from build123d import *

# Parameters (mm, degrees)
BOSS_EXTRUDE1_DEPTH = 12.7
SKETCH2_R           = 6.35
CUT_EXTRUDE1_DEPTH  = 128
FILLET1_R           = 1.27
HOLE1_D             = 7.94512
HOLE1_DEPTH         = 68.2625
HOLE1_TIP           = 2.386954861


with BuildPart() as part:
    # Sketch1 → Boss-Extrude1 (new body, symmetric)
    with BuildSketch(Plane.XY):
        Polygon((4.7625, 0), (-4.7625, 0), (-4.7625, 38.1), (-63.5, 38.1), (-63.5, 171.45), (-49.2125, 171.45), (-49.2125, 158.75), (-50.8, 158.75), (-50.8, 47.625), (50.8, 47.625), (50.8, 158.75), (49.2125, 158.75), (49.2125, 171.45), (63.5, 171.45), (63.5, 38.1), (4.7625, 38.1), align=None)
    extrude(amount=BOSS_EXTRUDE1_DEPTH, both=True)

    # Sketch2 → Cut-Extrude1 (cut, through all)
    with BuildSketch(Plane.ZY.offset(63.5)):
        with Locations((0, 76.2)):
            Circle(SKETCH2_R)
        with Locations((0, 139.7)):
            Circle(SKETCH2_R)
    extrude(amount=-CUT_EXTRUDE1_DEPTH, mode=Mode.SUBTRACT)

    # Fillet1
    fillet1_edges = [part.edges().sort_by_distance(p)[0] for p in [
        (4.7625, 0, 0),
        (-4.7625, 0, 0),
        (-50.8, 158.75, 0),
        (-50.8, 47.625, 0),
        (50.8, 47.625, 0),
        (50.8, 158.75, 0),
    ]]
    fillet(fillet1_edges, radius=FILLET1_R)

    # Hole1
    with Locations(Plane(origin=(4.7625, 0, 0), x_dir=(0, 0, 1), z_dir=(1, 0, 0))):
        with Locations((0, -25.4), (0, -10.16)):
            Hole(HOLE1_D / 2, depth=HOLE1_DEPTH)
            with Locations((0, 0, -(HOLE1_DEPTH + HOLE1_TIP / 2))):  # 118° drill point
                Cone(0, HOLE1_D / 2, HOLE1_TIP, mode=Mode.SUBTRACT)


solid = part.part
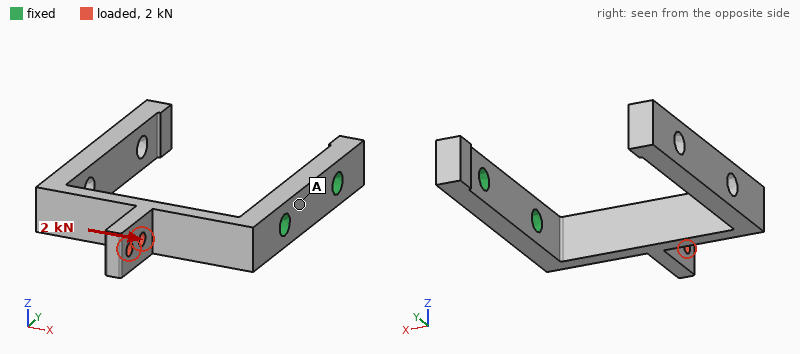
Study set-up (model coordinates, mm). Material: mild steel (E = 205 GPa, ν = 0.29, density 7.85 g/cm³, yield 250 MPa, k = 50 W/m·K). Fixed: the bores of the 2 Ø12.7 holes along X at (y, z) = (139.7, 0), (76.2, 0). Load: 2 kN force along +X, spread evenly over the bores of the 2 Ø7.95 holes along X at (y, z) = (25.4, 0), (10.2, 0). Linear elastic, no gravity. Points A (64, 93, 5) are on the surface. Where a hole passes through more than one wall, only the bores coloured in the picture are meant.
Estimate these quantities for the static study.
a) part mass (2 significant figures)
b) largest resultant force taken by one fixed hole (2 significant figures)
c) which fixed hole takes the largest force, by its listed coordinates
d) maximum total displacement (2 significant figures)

890 g
2.0 kN
(76.2, 0)
1.5 mm
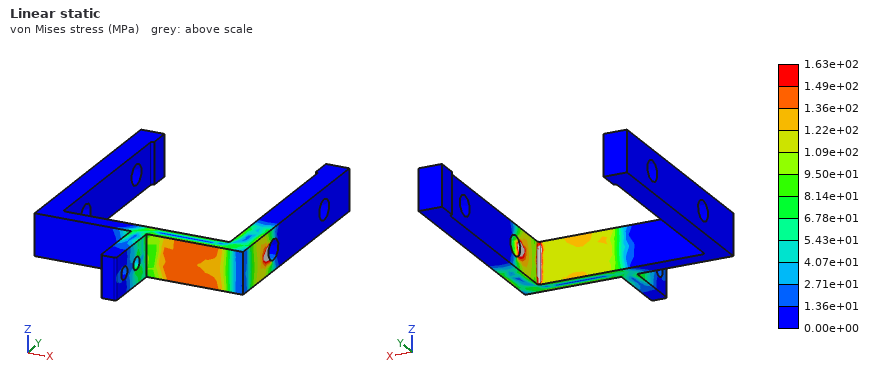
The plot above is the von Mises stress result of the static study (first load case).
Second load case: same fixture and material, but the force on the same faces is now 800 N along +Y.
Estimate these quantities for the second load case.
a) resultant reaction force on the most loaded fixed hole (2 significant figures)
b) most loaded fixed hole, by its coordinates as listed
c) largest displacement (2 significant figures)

790 N
(76.2, 0)
0.74 mm
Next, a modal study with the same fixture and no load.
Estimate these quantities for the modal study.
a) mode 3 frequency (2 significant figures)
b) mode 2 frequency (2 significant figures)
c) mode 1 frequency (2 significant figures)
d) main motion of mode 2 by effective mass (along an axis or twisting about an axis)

450 Hz
210 Hz
150 Hz
along Z
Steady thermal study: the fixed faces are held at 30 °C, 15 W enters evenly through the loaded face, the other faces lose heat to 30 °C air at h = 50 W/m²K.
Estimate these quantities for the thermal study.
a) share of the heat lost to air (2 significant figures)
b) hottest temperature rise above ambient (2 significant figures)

82 %
45 K
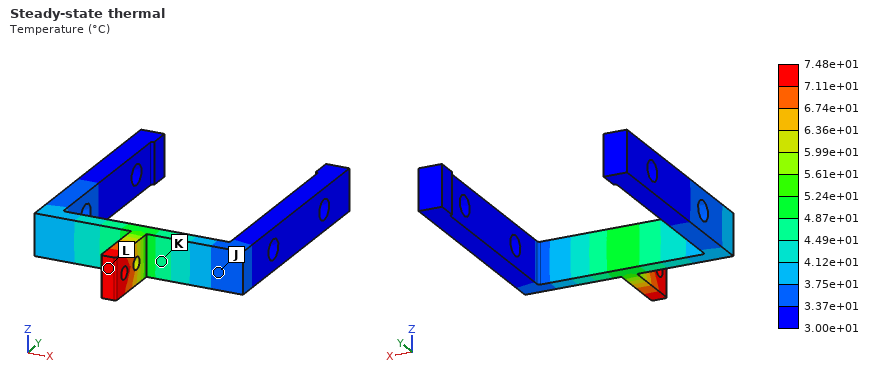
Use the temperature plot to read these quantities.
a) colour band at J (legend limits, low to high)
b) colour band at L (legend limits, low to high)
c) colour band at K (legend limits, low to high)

3.37e+01 to 3.75e+01 °C
7.11e+01 to 7.48e+01 °C
4.49e+01 to 4.87e+01 °C
